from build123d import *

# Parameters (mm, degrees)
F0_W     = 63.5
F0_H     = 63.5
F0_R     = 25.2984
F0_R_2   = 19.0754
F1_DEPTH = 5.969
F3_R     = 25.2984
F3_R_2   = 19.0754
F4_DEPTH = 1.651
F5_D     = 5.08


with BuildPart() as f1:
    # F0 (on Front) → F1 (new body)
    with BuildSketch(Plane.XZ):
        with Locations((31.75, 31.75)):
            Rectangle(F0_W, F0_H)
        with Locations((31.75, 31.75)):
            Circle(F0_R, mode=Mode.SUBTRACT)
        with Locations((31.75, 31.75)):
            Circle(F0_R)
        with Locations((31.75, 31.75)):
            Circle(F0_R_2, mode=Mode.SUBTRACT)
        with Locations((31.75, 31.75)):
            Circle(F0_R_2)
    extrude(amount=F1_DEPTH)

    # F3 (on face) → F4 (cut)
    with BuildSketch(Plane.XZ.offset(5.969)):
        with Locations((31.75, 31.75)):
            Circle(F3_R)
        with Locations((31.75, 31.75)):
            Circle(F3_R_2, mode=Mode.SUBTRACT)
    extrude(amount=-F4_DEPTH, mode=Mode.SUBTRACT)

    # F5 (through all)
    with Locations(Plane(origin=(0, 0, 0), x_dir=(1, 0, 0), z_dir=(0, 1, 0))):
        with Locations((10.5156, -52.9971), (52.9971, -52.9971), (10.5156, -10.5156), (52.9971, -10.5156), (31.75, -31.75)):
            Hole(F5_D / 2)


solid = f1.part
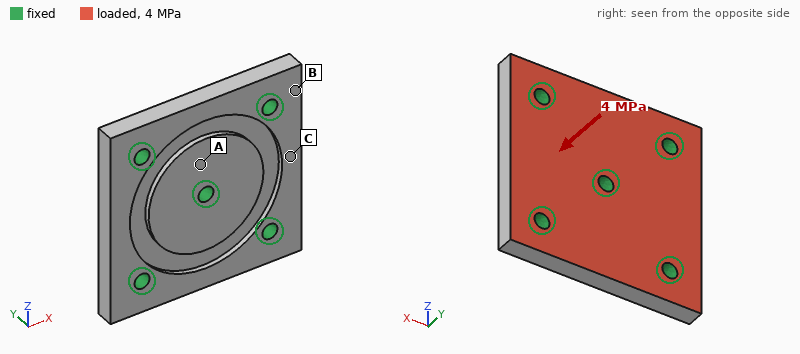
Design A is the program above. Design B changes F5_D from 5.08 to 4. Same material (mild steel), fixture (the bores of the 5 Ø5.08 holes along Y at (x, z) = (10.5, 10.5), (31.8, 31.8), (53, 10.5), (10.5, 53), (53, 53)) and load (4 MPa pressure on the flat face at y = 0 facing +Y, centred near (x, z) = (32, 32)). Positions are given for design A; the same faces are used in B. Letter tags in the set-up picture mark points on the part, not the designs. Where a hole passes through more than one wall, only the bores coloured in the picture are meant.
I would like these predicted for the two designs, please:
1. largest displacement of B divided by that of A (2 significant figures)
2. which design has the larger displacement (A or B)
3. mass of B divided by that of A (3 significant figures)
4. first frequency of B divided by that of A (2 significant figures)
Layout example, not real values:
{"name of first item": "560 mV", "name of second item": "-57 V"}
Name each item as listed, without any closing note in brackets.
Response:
{"largest displacement of B divided by that of A": "1.1", "which design has the larger displacement": "B", "mass of B divided by that of A": "1.01", "first frequency of B divided by that of A": "0.92"}
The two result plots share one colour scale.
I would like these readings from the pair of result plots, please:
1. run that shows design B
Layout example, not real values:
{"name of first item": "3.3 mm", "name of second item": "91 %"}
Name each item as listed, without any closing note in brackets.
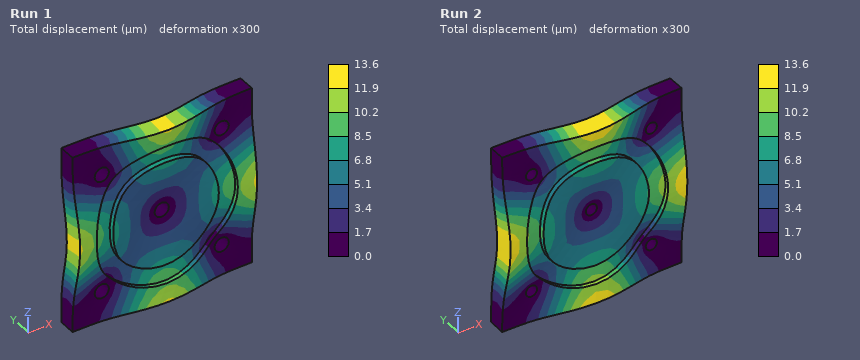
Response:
{"run that shows design B": "Run 2"}
